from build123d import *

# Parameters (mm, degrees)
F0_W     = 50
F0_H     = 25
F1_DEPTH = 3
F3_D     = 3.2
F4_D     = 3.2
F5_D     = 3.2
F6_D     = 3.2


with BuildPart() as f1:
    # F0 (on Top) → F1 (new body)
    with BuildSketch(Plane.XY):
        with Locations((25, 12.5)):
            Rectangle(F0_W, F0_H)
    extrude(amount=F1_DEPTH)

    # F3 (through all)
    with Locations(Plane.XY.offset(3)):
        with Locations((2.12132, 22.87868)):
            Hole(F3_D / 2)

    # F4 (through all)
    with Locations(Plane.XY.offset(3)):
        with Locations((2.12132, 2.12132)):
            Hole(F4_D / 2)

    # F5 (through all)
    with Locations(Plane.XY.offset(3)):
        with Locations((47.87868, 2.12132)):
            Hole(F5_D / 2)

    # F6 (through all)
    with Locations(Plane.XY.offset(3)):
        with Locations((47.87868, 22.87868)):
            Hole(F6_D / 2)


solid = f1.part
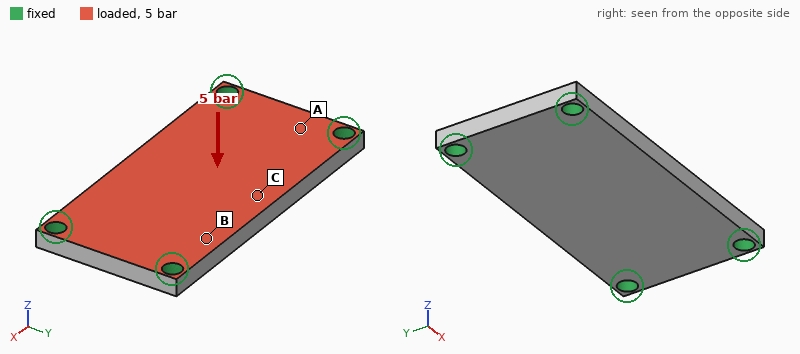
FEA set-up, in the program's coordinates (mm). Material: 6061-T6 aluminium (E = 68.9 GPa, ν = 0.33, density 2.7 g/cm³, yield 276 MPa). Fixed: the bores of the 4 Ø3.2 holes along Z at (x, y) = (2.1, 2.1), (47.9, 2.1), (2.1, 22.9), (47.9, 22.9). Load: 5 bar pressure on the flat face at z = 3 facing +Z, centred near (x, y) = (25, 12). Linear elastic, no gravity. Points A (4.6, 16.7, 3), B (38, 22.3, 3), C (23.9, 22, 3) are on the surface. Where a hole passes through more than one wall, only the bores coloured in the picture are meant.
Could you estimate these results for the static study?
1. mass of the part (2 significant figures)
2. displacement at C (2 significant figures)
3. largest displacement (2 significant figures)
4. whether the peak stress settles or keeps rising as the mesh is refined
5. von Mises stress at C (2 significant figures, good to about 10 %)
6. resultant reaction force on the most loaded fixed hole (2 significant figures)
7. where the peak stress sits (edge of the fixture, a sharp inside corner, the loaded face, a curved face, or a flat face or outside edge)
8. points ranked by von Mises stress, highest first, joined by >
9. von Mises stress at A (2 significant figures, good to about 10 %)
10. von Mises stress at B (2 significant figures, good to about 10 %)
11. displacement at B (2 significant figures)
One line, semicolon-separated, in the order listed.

9.9 g; 42 µm; 44 µm; keeps rising; 31 MPa; 150 N; edge of the fixture; C > A > B; 18 MPa; 10 MPa; 20 µm
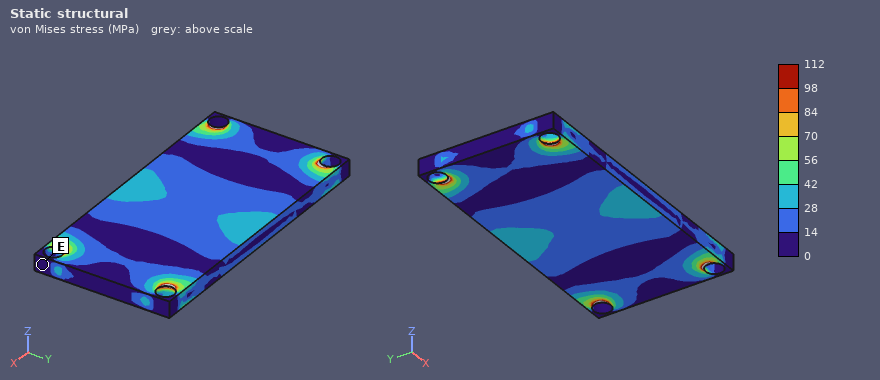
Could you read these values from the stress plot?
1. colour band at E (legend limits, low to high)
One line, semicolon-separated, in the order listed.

0 to 14 MPa
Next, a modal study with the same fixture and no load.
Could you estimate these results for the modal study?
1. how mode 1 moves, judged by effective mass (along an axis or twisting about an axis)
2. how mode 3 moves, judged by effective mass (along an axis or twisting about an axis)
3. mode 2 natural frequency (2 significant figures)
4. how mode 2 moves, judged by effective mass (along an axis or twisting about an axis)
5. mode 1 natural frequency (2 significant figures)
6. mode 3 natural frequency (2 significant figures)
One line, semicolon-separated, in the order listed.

along Z; twisting about Y; 12 kHz; twisting about X; 6900 Hz; 19 kHz
